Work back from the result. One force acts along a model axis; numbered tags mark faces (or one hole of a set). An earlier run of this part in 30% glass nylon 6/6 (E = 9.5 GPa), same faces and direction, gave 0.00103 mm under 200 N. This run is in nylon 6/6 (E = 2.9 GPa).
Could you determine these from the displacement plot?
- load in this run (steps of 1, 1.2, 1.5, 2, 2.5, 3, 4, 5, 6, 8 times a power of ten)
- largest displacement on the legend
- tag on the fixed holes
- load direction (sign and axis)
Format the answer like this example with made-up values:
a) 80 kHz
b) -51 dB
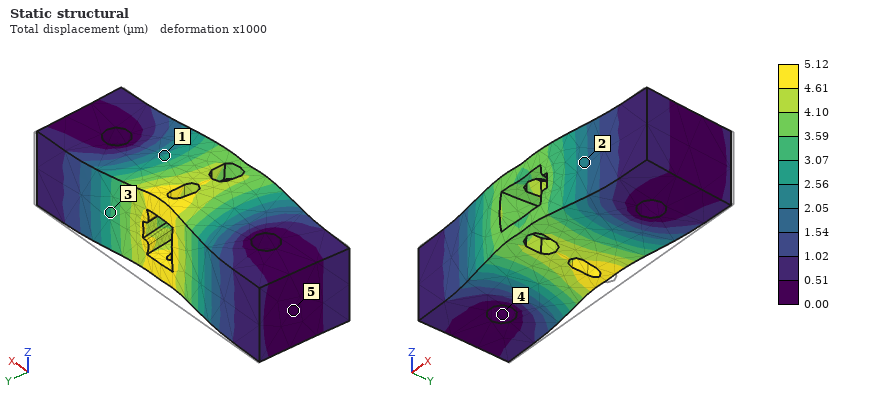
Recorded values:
a) 300 N
b) 5.12 µm
c) 4
d) -Y
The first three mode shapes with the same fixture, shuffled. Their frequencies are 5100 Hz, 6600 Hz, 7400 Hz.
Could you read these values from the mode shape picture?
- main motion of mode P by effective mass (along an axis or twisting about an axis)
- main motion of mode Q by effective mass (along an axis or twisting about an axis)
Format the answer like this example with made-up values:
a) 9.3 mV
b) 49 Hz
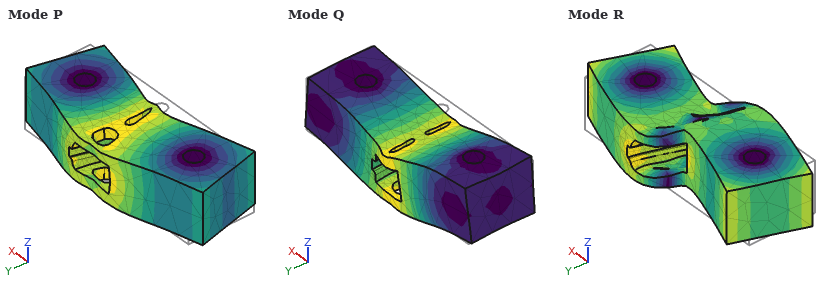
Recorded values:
a) along Y
b) along Z
